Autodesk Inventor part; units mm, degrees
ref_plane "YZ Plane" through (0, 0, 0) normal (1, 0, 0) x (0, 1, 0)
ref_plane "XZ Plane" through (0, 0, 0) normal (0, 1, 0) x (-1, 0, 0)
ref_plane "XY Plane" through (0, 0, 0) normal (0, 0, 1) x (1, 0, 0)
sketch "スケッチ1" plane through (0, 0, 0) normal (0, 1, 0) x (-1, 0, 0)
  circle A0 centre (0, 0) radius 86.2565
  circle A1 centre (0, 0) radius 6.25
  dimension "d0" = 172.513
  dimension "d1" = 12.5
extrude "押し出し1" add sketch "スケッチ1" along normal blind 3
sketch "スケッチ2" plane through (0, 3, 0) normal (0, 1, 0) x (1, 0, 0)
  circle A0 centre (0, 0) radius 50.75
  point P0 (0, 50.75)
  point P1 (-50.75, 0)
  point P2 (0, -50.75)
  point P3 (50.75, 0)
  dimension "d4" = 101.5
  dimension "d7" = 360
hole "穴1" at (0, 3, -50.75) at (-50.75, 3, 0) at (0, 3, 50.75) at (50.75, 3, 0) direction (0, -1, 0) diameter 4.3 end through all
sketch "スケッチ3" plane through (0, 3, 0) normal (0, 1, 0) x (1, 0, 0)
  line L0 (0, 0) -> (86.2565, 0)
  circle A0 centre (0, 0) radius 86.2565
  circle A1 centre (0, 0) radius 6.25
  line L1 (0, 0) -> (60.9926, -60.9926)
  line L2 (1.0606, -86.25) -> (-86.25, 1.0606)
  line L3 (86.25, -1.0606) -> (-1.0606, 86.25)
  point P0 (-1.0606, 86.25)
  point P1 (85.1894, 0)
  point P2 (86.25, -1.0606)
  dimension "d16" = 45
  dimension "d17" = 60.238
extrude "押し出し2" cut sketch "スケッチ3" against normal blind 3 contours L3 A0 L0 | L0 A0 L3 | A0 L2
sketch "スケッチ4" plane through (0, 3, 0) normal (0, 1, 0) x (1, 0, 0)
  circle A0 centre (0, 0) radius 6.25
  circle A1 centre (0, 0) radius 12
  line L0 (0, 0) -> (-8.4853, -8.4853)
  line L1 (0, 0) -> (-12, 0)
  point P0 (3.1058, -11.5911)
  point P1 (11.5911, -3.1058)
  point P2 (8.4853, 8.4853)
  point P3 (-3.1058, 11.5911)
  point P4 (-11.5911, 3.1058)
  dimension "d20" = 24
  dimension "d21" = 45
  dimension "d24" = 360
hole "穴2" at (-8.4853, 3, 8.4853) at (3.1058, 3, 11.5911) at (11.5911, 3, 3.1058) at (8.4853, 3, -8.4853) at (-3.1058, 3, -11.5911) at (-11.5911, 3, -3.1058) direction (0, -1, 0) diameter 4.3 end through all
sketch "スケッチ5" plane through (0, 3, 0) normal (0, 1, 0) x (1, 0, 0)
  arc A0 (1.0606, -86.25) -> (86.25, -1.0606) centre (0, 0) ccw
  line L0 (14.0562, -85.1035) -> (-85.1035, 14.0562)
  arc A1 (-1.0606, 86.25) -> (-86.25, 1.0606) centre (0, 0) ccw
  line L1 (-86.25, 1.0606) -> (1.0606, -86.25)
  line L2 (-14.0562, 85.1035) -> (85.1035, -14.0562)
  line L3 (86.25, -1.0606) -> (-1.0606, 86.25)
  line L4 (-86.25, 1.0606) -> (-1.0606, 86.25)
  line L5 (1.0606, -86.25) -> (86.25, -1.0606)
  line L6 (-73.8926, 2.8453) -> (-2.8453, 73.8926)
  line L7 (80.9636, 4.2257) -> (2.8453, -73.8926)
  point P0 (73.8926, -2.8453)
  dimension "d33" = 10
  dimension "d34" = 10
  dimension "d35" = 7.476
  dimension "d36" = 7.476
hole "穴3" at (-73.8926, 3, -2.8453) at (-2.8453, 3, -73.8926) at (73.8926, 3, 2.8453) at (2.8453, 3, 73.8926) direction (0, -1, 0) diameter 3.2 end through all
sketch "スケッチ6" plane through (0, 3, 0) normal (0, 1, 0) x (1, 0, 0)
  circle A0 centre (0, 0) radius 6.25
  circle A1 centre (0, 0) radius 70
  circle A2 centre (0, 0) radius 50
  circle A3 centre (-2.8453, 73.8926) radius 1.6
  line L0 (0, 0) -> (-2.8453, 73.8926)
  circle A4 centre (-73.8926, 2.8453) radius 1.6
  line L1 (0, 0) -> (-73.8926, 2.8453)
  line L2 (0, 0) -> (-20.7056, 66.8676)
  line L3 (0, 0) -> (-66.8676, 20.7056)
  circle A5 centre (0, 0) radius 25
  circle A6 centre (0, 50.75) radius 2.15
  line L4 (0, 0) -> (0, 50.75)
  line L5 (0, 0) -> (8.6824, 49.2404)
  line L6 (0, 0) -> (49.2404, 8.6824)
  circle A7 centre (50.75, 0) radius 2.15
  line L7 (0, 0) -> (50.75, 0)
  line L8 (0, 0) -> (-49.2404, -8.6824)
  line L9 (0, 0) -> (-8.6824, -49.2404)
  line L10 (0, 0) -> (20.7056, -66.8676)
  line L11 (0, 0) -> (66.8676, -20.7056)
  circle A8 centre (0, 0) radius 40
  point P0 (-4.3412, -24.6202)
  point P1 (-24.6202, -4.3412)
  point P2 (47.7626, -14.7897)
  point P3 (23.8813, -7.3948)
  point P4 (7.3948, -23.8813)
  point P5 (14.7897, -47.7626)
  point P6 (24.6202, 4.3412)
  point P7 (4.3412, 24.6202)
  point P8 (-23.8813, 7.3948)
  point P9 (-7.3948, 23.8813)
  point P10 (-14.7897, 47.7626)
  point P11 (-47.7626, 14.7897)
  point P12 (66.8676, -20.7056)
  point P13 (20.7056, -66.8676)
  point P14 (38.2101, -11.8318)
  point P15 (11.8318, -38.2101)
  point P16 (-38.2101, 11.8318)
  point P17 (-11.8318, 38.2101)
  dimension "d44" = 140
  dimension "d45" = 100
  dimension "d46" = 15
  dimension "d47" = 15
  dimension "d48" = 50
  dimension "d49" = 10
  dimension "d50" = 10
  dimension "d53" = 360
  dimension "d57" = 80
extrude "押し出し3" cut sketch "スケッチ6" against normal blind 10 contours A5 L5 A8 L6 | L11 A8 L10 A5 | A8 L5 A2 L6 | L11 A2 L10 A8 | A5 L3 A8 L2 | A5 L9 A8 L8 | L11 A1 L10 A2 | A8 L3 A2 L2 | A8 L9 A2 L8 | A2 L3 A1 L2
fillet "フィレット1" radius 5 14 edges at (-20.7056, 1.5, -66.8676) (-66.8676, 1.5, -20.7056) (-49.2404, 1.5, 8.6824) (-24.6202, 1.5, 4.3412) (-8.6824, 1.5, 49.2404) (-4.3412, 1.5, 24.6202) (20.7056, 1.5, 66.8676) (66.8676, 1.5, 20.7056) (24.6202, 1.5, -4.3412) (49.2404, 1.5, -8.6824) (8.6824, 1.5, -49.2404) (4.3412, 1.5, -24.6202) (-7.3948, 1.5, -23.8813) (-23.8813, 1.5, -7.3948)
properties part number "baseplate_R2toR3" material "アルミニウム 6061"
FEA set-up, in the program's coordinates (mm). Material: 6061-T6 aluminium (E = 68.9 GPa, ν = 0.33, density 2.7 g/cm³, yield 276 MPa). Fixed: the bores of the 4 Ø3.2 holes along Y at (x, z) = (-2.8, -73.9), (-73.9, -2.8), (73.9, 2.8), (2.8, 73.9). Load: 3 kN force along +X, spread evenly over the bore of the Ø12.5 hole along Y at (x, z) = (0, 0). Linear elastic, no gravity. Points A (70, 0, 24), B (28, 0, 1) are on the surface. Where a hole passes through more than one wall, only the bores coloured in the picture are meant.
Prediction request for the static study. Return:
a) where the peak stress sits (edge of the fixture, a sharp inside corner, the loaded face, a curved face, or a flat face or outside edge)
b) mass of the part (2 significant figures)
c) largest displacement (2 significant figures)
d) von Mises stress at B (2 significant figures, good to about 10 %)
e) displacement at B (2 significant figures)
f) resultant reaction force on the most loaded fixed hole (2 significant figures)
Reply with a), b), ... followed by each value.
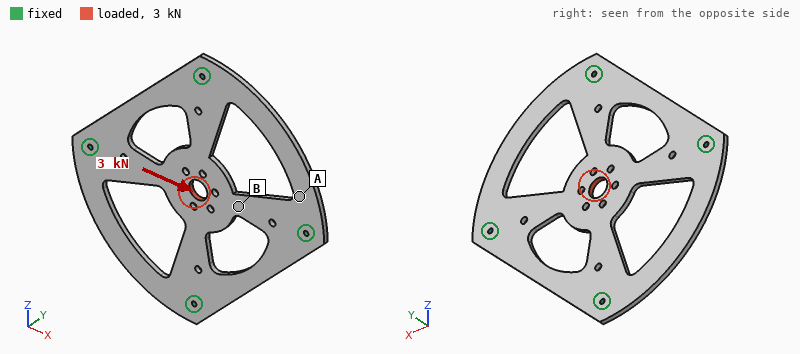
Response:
a) a curved face
b) 99 g
c) 29 µm
d) 26 MPa
e) 17 µm
f) 1.3 kN
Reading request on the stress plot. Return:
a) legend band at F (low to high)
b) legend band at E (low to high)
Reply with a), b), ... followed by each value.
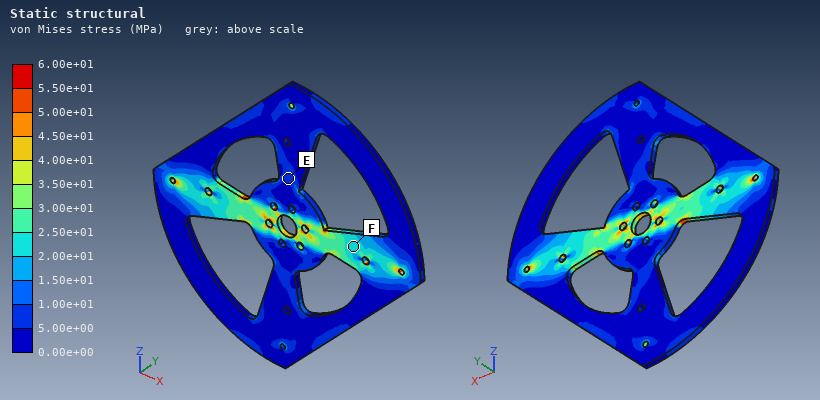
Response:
a) 2.00e+01 to 2.50e+01 MPa
b) 5.00e+00 to 1.00e+01 MPa
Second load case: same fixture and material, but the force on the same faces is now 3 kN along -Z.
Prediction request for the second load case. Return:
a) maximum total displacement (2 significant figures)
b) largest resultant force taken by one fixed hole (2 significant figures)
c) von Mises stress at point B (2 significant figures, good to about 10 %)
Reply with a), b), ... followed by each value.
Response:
a) 29 µm
b) 1.3 kN
c) 7.6 MPa
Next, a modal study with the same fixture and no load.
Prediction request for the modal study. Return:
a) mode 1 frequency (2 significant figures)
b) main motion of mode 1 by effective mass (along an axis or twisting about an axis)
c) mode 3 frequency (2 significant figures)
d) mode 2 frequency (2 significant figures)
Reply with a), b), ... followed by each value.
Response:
a) 900 Hz
b) along Y
c) 1200 Hz
d) 1200 Hz
